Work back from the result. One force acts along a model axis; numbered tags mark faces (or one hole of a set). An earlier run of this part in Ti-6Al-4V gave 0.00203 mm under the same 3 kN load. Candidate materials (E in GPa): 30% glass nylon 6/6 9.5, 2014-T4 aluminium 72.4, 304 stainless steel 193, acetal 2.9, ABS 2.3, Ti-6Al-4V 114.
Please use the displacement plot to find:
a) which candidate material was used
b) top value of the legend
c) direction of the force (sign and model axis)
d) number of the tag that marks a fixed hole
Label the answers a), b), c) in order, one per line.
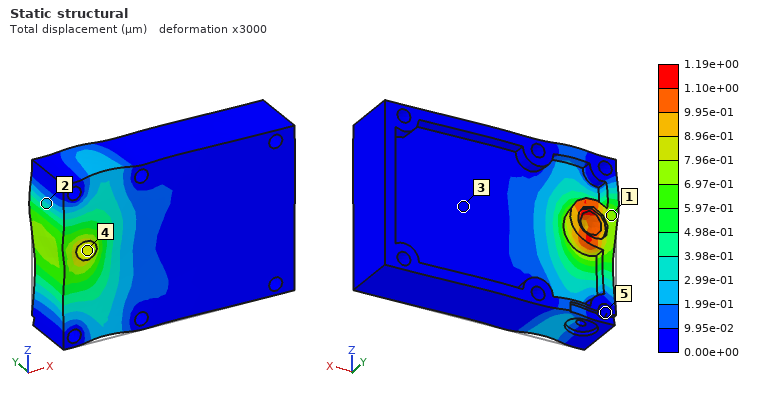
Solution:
a) 304 stainless steel
b) 1.19e+00 µm
c) +Z
d) 5
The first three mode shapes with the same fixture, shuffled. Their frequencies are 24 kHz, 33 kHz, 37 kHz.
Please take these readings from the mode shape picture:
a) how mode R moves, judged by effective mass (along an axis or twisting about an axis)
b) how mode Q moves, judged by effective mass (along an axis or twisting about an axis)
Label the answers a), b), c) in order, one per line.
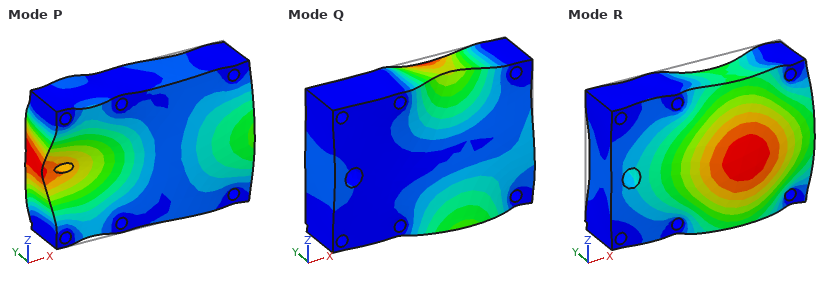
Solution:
a) along Y
b) along Z
